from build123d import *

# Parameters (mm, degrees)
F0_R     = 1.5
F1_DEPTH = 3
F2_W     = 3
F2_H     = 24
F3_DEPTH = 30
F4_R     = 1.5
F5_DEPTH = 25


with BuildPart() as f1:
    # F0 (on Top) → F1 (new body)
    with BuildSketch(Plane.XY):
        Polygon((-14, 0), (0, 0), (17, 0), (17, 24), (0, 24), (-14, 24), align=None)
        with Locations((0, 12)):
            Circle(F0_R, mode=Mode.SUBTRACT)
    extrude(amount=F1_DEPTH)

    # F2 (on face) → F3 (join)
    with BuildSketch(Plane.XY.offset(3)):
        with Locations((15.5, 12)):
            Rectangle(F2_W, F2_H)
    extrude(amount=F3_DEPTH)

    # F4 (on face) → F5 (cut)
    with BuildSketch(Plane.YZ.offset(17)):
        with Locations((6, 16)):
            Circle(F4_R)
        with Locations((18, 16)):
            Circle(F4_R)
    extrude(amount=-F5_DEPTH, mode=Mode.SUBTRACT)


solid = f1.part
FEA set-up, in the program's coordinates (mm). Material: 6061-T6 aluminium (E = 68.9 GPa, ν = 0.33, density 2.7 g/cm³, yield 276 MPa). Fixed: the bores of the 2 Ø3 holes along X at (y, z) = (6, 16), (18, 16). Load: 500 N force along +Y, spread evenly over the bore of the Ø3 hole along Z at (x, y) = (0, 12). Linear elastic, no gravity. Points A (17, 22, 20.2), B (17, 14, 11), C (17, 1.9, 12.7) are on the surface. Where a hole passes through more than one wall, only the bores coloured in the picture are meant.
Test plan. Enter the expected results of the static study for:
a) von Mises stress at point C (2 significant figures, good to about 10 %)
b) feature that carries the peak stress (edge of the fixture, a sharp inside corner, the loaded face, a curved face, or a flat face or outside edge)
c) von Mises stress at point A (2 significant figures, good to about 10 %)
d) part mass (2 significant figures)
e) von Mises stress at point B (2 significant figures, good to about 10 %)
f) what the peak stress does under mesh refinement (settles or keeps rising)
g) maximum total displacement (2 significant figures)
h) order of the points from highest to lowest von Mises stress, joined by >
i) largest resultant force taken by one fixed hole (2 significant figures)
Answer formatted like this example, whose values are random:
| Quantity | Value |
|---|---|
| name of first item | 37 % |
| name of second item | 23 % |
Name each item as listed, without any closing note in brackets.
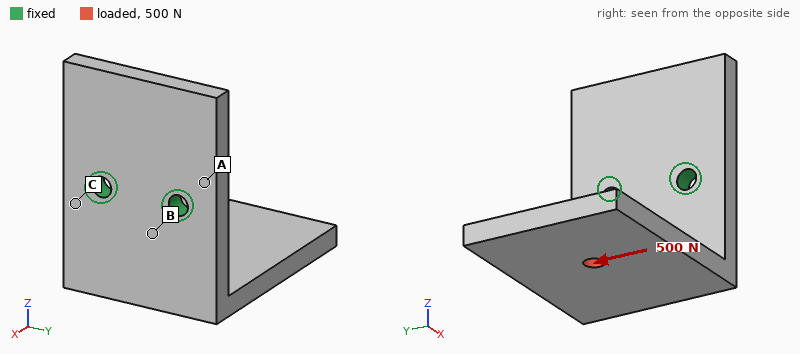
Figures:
| Quantity | Value |
|---|---|
| von Mises stress at point C | 120 MPa |
| feature that carries the peak stress | edge of the fixture |
| von Mises stress at point A | 29 MPa |
| part mass | 12 g |
| von Mises stress at point B | 81 MPa |
| what the peak stress does under mesh refinement | keeps rising |
| maximum total displacement | 0.34 mm |
| order of the points from highest to lowest von Mises stress, joined by > | C > B > A |
| largest resultant force taken by one fixed hole | 750 N |
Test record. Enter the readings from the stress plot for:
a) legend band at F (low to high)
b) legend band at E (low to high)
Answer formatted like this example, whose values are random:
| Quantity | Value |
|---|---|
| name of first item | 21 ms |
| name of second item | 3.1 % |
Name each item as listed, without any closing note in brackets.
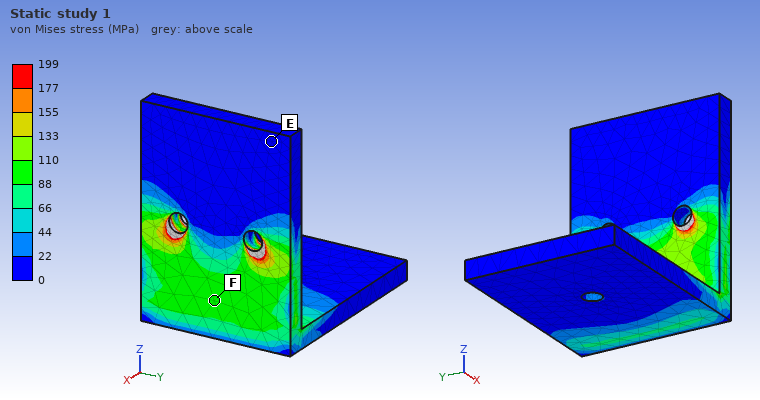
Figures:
| Quantity | Value |
|---|---|
| legend band at F | 88 to 110 MPa |
| legend band at E | 0 to 22 MPa |
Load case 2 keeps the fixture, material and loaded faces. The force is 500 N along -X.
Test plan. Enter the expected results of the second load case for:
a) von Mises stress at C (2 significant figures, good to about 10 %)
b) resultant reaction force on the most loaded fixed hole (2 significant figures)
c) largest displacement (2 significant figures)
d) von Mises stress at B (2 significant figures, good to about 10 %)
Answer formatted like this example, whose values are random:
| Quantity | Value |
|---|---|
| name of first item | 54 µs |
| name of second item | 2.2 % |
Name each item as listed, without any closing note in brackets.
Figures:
| Quantity | Value |
|---|---|
| von Mises stress at C | 130 MPa |
| resultant reaction force on the most loaded fixed hole | 250 N |
| largest displacement | 0.41 mm |
| von Mises stress at B | 110 MPa |
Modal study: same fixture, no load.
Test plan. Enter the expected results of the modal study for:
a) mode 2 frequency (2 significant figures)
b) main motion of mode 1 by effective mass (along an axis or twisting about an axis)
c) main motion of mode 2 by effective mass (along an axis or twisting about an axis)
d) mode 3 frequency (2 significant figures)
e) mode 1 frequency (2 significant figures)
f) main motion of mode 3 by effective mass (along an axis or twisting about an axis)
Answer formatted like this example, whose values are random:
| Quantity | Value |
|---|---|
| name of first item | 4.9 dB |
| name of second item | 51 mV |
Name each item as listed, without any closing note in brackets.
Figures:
| Quantity | Value |
|---|---|
| mode 2 frequency | 3000 Hz |
| main motion of mode 1 by effective mass | along Z |
| main motion of mode 2 by effective mass | along Y |
| mode 3 frequency | 5700 Hz |
| mode 1 frequency | 1600 Hz |
| main motion of mode 3 by effective mass | along X |
